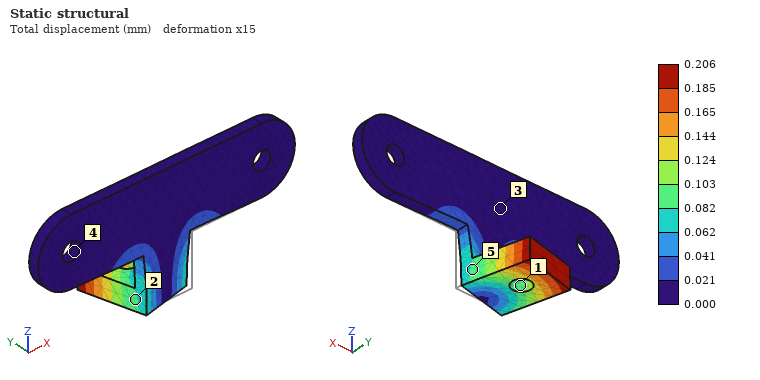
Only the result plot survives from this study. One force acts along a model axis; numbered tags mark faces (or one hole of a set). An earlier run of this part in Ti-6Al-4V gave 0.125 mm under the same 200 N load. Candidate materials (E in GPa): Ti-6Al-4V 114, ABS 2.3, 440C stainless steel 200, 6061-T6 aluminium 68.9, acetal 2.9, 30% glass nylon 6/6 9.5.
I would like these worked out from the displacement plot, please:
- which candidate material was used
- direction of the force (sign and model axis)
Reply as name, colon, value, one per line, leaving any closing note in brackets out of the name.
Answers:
which candidate material was used: 6061-T6 aluminium
direction of the force: -X
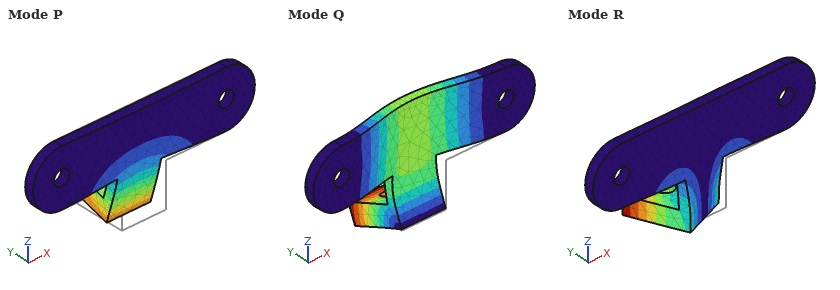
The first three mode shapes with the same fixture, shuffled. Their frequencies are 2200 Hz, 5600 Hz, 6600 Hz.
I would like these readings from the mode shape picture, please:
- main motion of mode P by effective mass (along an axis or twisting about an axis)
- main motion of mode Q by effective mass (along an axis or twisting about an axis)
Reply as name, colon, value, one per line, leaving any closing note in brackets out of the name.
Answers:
main motion of mode P by effective mass: along Y
main motion of mode Q by effective mass: along Y
